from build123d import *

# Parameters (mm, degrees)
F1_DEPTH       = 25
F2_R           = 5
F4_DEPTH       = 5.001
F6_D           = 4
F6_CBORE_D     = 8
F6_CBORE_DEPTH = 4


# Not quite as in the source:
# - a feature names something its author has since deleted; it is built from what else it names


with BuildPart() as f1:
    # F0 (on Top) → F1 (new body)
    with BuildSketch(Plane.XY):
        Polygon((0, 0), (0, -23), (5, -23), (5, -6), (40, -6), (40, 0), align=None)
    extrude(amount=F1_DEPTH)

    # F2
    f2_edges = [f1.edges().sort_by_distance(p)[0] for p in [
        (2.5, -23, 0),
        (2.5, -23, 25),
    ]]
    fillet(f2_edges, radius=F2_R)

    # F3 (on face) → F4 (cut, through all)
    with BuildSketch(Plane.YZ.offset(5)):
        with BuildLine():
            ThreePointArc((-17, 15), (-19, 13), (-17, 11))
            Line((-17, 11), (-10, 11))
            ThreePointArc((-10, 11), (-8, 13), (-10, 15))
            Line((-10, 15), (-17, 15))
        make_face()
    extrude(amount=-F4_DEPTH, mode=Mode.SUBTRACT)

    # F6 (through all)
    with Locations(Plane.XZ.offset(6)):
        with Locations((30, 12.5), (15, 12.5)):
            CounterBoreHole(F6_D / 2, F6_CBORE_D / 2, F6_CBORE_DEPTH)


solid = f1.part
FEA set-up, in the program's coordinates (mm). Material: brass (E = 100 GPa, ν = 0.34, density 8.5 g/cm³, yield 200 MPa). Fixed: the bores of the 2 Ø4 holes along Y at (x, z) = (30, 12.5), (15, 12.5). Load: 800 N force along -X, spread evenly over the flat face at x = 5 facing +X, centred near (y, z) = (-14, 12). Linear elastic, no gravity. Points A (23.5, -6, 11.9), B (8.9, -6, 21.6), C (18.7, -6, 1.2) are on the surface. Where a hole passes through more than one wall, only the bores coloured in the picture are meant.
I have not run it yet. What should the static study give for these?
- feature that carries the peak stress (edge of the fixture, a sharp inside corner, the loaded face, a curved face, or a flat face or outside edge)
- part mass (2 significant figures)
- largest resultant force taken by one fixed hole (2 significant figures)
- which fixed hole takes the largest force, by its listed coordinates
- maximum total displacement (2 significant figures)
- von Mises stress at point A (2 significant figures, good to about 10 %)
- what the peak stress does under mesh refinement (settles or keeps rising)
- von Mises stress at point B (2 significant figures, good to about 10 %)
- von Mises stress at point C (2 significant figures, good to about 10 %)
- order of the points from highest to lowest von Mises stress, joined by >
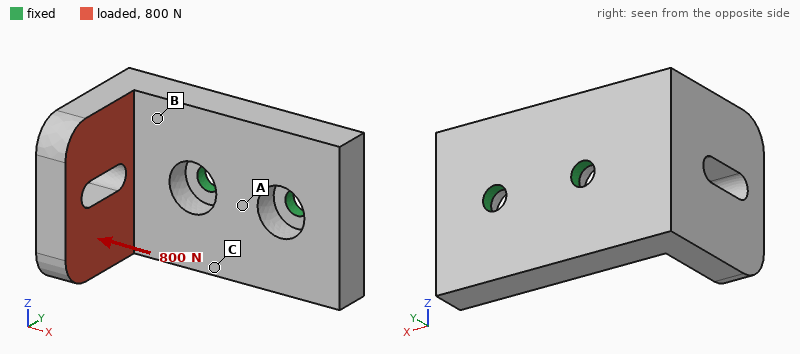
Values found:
edge of the fixture
63 g
1.1 kN
(30, 12.5)
0.12 mm
13 MPa
keeps rising
74 MPa
47 MPa
B > C > A
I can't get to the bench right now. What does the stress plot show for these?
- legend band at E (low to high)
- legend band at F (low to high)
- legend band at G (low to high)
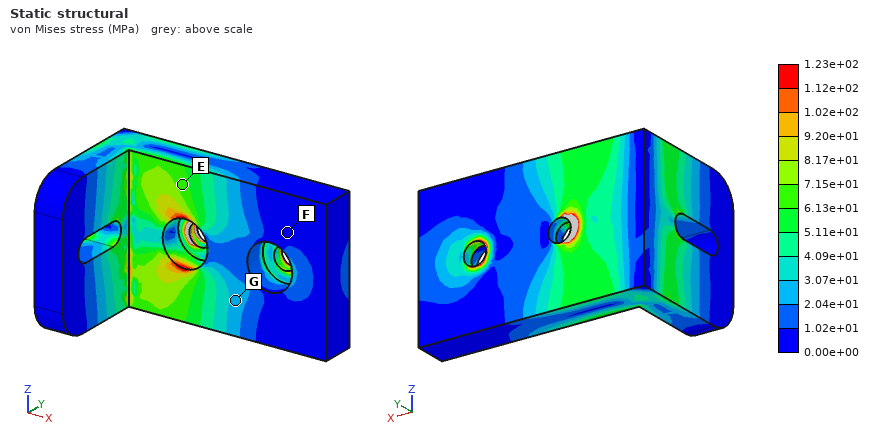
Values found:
6.13e+01 to 7.15e+01 MPa
0.00e+00 to 1.02e+01 MPa
2.04e+01 to 3.07e+01 MPa
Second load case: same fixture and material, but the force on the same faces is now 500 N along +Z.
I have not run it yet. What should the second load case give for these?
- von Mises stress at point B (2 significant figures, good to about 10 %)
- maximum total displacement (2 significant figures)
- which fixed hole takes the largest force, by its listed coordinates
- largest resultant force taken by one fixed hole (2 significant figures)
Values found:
26 MPa
92 µm
(15, 12.5)
710 N
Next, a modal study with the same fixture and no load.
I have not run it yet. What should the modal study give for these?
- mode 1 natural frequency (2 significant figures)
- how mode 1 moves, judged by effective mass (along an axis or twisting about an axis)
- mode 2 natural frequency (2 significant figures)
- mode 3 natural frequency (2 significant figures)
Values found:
2900 Hz
along Z
3400 Hz
8200 Hz
